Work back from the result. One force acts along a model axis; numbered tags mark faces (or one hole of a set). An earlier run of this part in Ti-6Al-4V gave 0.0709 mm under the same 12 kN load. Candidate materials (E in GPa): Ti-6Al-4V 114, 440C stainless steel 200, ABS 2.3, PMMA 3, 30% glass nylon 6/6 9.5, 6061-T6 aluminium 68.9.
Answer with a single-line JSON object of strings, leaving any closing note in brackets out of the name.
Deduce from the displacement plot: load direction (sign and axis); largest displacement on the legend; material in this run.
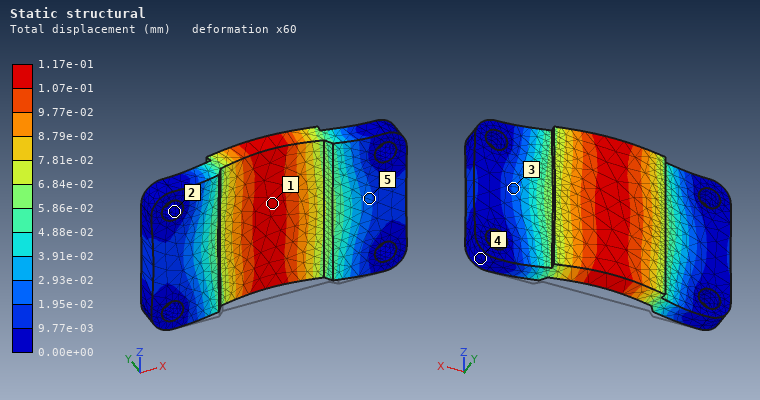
{"load direction": "+Y", "largest displacement on the legend": "1.17e-01 mm", "material in this run": "6061-T6 aluminium"}
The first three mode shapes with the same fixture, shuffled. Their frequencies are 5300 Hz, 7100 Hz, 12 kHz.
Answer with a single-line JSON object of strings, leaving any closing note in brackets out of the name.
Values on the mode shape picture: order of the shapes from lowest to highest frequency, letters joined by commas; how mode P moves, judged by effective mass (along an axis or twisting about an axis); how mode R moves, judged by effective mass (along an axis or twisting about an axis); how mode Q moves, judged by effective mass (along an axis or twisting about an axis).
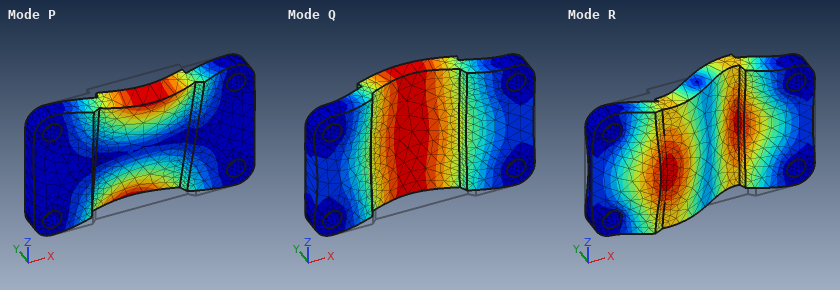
{"order of the shapes from lowest to highest frequency, letters joined by commas": "Q, P, R", "how mode P moves, judged by effective mass": "twisting about X", "how mode R moves, judged by effective mass": "twisting about Z", "how mode Q moves, judged by effective mass": "along Y"}
